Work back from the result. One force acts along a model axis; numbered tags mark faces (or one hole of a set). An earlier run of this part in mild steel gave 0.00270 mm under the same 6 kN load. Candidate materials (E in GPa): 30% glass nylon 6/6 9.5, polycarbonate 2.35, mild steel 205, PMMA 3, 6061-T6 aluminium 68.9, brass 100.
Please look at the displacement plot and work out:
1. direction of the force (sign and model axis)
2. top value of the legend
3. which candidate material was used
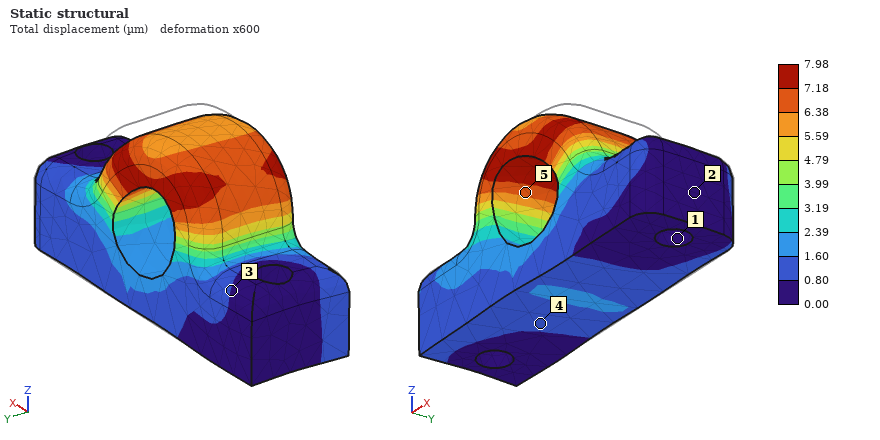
-X
7.98 µm
6061-T6 aluminium
